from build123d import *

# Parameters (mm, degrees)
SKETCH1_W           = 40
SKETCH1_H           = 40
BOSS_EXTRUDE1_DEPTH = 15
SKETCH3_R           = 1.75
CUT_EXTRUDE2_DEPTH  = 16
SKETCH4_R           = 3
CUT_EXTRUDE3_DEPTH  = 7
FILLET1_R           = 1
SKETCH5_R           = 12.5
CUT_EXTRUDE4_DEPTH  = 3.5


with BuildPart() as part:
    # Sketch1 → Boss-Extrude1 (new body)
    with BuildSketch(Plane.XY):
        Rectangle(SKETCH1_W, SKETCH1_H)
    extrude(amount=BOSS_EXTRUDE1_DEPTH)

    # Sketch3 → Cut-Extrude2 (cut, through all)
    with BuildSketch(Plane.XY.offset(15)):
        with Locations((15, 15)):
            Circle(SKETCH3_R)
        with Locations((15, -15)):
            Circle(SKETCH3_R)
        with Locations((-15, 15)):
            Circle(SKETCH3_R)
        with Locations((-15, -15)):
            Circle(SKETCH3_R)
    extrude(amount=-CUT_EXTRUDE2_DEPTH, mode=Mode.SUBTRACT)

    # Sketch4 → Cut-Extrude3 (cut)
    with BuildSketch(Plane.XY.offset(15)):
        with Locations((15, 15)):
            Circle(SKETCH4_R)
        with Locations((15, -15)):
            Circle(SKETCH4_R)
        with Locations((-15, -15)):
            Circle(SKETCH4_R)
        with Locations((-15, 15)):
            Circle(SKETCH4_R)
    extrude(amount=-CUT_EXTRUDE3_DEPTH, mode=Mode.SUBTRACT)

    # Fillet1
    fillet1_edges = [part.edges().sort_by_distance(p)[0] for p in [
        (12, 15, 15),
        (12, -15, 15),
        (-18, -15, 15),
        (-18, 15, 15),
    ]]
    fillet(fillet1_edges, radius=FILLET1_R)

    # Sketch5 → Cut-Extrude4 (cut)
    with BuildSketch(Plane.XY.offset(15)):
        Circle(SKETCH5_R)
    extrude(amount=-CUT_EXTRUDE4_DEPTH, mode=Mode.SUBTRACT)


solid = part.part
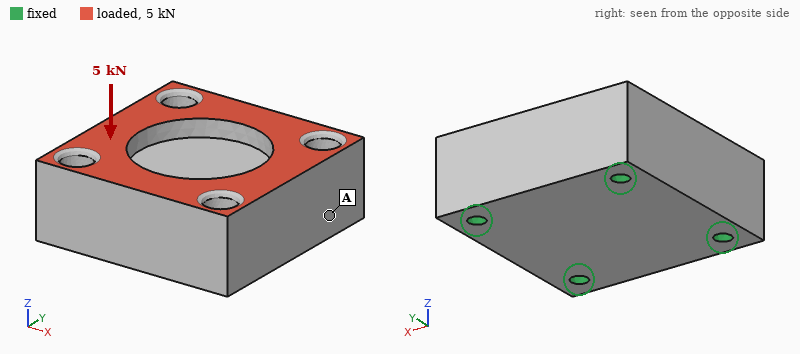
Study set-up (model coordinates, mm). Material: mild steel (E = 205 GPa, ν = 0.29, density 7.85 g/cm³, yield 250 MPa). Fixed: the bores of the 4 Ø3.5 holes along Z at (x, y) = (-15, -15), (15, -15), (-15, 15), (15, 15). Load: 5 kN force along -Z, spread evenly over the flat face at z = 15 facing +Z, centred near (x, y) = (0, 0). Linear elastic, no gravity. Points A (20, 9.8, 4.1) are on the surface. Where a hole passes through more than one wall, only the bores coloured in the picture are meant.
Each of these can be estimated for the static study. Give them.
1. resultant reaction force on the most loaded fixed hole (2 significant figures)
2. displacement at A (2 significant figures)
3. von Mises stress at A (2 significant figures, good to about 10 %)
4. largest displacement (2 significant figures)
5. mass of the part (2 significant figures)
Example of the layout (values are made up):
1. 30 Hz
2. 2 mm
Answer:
1. 1.3 kN
2. 0.52 µm
3. 7.8 MPa
4. 1.1 µm
5. 170 g
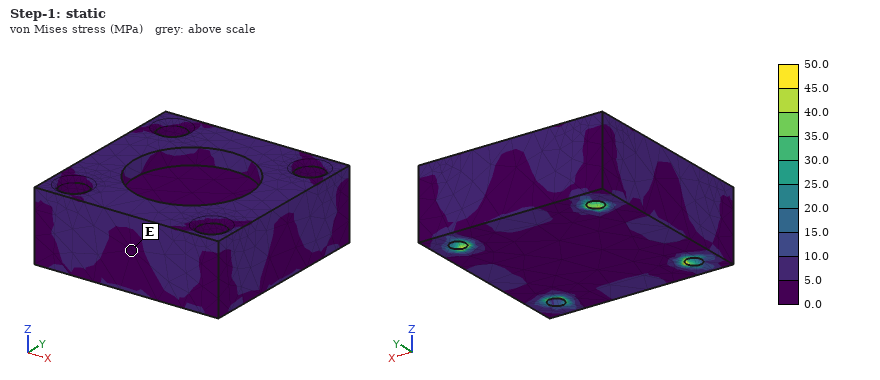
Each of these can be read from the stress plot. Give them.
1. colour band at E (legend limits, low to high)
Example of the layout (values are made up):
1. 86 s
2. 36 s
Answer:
1. 0.0 to 5.0 MPa
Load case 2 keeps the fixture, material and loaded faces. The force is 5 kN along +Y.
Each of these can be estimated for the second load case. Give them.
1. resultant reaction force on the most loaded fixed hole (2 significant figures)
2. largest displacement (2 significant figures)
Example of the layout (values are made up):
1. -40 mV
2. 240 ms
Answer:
1. 1.5 kN
2. 2.6 µm
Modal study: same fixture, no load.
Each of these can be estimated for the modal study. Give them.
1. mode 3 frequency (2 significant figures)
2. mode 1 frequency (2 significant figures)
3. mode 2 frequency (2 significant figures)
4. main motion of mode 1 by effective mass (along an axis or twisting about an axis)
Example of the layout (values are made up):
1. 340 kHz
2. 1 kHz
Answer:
1. 35 kHz
2. 27 kHz
3. 35 kHz
4. along Z
